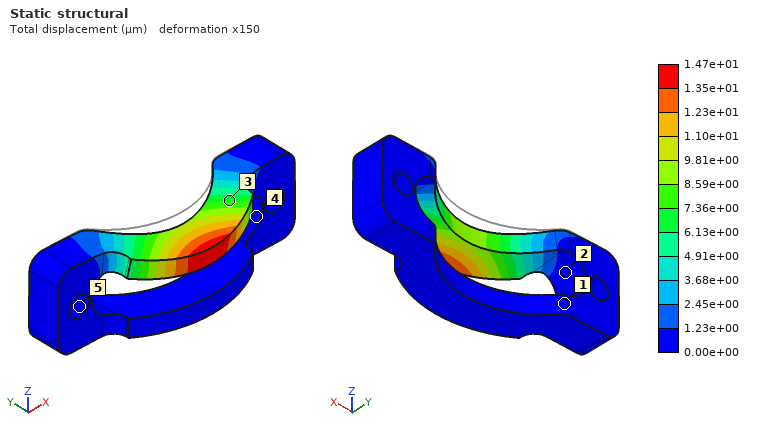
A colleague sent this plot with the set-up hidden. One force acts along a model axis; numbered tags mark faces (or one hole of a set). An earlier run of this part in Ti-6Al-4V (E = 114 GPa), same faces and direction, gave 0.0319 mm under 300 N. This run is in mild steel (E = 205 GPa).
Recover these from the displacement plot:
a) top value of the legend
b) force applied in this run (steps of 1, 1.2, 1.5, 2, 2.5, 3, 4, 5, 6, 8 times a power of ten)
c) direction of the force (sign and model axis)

1.47e+01 µm
250 N
-Z
